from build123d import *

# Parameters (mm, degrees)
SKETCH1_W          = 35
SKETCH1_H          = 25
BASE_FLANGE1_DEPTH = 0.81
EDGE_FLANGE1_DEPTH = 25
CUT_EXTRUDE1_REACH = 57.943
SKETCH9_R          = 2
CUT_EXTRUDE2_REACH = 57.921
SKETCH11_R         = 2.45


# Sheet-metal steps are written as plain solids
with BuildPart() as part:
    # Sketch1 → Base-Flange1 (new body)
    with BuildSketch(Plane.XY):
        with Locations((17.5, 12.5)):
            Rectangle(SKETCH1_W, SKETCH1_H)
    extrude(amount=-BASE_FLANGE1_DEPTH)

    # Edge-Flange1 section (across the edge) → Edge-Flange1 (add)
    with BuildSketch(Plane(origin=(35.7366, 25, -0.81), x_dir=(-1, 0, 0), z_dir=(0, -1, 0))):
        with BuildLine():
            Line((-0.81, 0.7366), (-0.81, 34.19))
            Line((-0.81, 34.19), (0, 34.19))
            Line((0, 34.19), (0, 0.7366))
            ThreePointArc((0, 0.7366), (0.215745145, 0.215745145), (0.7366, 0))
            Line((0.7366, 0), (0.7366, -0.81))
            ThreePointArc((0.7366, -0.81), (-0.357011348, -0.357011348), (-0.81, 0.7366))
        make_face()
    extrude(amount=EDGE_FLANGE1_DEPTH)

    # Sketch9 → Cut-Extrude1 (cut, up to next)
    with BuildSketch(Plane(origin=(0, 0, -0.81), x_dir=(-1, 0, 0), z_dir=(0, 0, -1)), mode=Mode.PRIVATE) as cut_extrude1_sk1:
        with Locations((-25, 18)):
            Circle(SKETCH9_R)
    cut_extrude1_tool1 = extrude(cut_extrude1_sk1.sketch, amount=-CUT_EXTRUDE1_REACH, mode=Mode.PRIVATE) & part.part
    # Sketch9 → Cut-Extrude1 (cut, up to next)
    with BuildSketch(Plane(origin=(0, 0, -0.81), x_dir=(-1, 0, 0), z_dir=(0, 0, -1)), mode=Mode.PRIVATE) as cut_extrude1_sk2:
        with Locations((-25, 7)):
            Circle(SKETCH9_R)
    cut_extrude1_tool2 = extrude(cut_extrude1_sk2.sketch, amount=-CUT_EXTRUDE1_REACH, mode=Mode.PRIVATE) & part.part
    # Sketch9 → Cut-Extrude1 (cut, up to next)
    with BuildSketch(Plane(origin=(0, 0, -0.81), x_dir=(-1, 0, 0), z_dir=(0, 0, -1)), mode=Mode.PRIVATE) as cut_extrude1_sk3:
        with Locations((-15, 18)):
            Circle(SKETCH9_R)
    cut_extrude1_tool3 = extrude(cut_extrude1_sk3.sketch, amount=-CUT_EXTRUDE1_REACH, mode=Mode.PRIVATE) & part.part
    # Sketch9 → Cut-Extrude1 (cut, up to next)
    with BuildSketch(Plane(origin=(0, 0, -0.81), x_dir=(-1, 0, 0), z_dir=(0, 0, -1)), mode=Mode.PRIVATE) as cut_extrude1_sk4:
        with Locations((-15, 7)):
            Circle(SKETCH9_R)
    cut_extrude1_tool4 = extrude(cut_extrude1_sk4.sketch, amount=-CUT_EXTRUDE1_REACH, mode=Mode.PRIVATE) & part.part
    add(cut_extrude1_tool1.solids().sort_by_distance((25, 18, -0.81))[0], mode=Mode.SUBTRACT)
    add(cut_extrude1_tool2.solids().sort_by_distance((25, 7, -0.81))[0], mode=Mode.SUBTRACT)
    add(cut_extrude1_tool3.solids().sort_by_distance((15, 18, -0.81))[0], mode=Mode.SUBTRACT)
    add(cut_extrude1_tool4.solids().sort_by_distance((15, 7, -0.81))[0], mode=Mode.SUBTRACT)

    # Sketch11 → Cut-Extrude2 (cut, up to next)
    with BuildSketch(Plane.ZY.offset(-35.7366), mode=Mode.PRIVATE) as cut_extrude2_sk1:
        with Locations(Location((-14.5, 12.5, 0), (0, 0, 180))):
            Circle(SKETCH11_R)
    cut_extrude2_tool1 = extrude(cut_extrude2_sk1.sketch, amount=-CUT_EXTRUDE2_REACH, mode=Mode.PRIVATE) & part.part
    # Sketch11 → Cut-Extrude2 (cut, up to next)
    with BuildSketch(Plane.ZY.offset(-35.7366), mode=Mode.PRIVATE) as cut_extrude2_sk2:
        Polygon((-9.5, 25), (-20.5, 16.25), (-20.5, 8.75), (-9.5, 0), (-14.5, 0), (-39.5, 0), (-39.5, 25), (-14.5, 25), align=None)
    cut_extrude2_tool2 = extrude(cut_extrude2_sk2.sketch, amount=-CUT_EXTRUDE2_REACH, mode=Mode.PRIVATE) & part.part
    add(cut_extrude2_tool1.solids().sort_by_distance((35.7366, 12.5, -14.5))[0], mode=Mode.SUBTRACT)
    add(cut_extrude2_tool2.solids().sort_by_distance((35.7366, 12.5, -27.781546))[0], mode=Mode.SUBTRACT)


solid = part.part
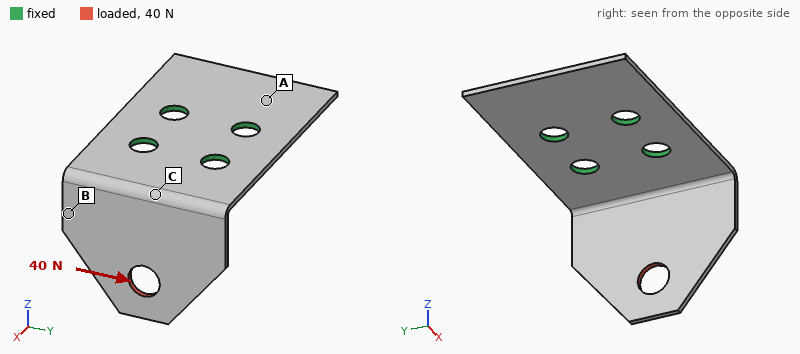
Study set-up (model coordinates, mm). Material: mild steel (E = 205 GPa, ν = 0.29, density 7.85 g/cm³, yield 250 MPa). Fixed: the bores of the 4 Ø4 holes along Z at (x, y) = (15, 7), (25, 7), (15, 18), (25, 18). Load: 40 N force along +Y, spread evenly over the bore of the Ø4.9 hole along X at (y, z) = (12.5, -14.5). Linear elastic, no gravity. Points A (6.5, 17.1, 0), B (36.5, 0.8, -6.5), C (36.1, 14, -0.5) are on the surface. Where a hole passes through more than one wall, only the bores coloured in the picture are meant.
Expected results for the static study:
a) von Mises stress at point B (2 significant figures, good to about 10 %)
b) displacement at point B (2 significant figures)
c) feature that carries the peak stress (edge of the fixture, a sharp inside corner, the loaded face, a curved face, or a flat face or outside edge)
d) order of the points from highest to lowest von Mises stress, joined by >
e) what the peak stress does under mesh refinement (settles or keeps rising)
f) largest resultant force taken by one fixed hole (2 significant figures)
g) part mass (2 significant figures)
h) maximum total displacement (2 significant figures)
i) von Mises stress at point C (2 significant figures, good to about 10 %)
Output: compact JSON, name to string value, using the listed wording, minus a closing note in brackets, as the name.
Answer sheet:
{"von Mises stress at point B": "34 MPa", "displacement at point B": "0.085 mm", "feature that carries the peak stress": "edge of the fixture", "order of the points from highest to lowest von Mises stress, joined by >": "C > B > A", "what the peak stress does under mesh refinement": "keeps rising", "largest resultant force taken by one fixed hole": "49 N", "part mass": "7.8 g", "maximum total displacement": "0.13 mm", "von Mises stress at point C": "61 MPa"}
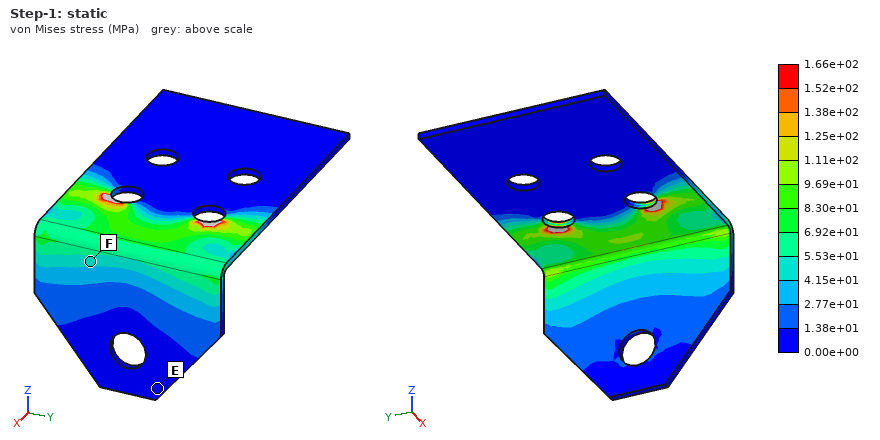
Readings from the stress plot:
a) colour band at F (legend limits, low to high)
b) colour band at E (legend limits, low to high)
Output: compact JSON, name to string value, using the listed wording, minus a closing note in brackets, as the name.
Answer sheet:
{"colour band at F": "4.15e+01 to 5.53e+01 MPa", "colour band at E": "0.00e+00 to 1.38e+01 MPa"}
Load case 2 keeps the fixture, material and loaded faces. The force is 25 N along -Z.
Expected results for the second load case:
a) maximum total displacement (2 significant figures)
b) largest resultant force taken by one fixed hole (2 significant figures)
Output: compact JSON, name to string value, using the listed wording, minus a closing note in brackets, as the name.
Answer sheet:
{"maximum total displacement": "0.11 mm", "largest resultant force taken by one fixed hole": "13 N"}
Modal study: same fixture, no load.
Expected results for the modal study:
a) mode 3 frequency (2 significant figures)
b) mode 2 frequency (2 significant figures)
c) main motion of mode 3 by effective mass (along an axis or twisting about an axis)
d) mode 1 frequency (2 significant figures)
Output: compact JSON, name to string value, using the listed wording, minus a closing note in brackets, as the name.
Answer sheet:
{"mode 3 frequency": "3600 Hz", "mode 2 frequency": "2500 Hz", "main motion of mode 3 by effective mass": "along Z", "mode 1 frequency": "1300 Hz"}
